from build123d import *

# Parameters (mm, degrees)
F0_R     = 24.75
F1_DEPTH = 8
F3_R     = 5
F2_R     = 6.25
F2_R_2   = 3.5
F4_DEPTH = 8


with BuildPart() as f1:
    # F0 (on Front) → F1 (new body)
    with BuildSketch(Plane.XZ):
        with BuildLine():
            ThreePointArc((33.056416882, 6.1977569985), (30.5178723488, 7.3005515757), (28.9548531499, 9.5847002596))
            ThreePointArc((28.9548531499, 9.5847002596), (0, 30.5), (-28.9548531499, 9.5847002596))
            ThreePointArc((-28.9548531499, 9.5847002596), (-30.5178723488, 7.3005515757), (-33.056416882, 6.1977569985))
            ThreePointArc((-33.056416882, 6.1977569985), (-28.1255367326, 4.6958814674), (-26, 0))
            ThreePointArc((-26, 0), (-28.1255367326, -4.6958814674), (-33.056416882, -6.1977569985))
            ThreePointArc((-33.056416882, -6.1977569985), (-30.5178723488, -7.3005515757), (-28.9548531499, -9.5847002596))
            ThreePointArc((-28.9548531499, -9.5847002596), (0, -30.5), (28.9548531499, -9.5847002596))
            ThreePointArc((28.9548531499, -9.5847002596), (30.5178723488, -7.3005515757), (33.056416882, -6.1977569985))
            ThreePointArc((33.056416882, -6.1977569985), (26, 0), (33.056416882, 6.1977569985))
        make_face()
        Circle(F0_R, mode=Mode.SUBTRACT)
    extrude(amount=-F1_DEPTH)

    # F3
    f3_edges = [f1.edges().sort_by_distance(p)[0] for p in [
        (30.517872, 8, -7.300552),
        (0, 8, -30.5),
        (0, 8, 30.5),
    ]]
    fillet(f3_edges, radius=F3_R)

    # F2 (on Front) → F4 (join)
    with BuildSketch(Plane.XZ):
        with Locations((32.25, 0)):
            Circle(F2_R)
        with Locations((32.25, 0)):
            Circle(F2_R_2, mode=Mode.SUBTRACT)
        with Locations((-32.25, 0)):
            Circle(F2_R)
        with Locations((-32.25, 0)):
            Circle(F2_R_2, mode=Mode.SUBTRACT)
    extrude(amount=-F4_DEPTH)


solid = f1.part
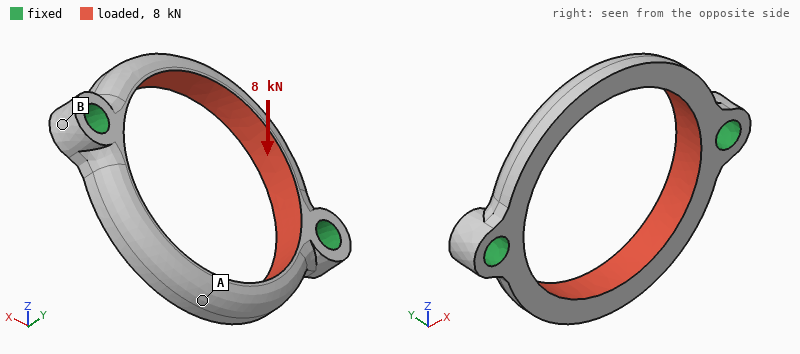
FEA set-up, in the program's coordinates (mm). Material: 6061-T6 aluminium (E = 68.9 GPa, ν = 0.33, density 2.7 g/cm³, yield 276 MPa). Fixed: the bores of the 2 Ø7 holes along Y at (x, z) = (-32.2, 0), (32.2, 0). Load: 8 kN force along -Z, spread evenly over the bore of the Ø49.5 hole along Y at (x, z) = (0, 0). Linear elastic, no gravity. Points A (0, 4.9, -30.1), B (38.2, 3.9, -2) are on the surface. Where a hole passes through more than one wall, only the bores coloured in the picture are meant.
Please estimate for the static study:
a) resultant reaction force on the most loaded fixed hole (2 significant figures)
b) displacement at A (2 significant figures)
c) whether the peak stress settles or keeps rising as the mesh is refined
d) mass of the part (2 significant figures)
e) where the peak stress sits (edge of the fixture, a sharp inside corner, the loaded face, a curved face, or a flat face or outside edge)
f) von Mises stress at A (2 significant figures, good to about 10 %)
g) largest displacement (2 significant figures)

4.0 kN
43 µm
keeps rising
21 g
edge of the fixture
54 MPa
46 µm
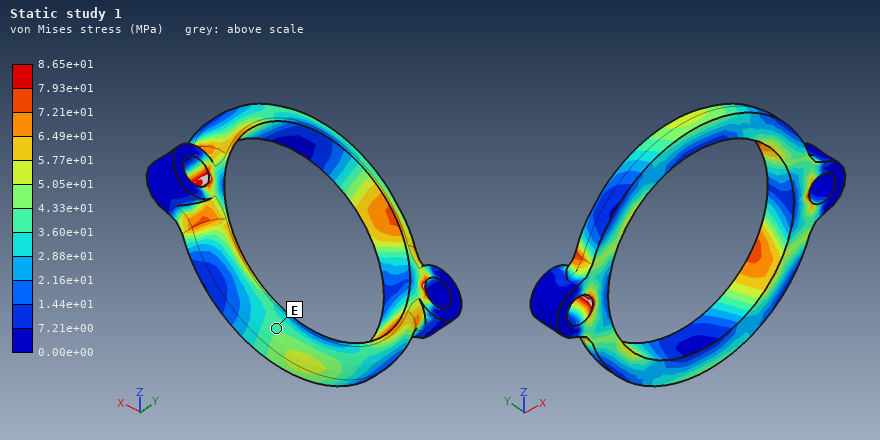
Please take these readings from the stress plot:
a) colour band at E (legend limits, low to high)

3.60e+01 to 4.33e+01 MPa
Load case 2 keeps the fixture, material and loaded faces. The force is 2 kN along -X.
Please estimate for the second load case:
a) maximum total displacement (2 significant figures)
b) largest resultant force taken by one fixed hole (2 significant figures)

36 µm
1.0 kN
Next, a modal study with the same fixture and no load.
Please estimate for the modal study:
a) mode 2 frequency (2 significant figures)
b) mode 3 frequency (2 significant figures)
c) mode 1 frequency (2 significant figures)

4700 Hz
8600 Hz
4500 Hz
